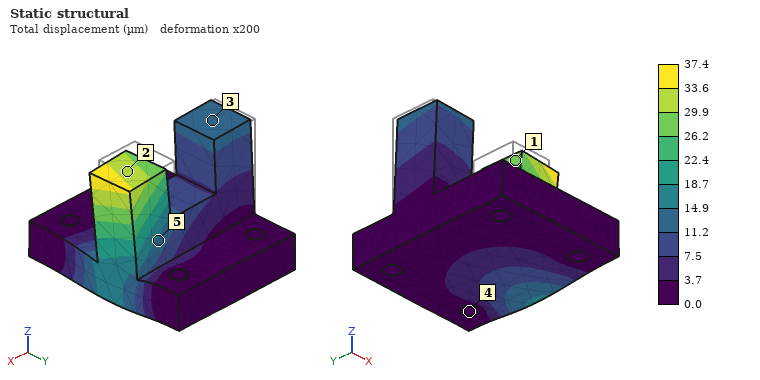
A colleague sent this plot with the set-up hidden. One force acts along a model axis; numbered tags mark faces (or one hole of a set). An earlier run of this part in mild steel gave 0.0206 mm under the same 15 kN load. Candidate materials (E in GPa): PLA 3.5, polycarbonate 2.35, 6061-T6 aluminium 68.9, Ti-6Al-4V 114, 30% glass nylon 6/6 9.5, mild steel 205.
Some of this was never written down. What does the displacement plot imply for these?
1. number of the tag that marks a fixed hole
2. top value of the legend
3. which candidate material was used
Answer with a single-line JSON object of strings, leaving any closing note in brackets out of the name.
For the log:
{"number of the tag that marks a fixed hole": "4", "top value of the legend": "37.4 µm", "which candidate material was used": "Ti-6Al-4V"}
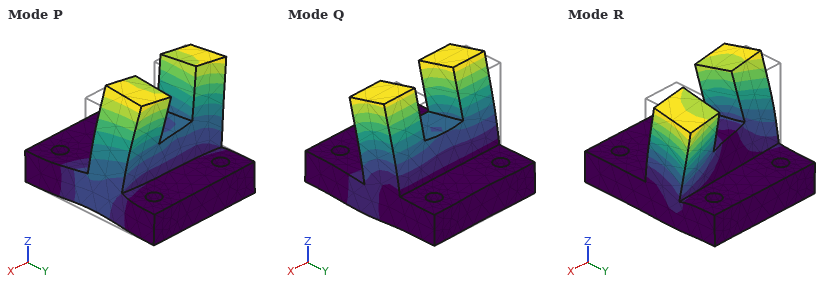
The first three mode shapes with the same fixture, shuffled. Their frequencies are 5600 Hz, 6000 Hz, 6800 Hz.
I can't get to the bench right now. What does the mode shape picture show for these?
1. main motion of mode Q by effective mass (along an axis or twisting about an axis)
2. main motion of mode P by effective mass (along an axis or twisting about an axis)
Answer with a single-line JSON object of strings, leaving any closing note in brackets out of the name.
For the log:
{"main motion of mode Q by effective mass": "along Y", "main motion of mode P by effective mass": "along X"}
